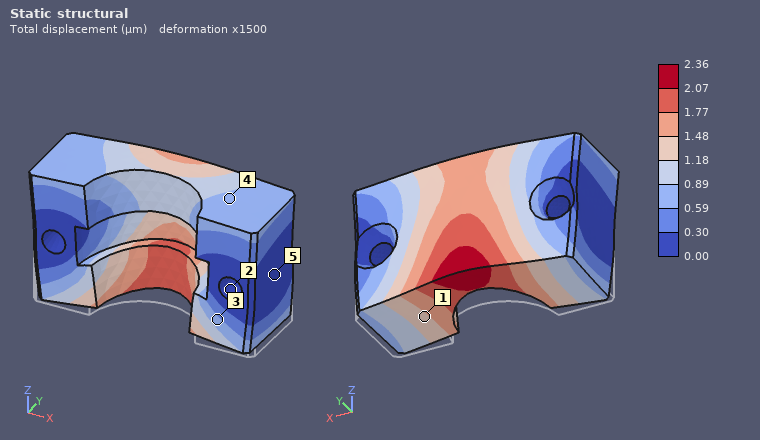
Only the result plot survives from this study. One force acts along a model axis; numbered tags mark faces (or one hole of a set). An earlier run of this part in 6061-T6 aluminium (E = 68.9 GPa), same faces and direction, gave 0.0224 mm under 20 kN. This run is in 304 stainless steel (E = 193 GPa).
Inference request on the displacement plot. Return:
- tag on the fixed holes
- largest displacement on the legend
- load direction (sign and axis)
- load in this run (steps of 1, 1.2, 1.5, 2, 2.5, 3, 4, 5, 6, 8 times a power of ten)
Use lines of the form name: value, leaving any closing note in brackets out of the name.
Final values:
tag on the fixed holes: 2
largest displacement on the legend: 2.36 µm
load direction: +Z
load in this run: 6 kN
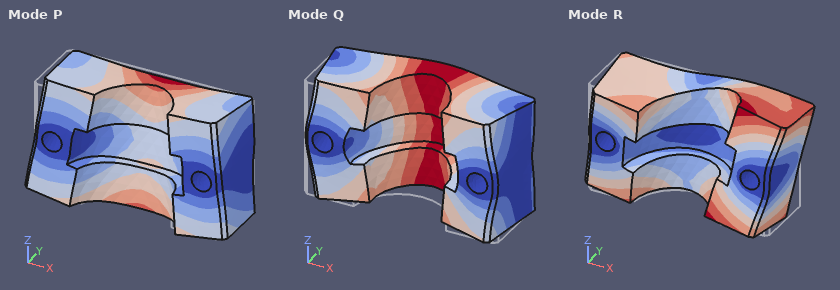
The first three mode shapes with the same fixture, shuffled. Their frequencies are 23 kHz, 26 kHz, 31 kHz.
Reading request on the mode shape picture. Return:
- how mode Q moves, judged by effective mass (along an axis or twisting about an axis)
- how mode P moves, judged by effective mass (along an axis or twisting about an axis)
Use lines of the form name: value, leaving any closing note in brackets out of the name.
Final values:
how mode Q moves, judged by effective mass: along Y
how mode P moves, judged by effective mass: along Z
